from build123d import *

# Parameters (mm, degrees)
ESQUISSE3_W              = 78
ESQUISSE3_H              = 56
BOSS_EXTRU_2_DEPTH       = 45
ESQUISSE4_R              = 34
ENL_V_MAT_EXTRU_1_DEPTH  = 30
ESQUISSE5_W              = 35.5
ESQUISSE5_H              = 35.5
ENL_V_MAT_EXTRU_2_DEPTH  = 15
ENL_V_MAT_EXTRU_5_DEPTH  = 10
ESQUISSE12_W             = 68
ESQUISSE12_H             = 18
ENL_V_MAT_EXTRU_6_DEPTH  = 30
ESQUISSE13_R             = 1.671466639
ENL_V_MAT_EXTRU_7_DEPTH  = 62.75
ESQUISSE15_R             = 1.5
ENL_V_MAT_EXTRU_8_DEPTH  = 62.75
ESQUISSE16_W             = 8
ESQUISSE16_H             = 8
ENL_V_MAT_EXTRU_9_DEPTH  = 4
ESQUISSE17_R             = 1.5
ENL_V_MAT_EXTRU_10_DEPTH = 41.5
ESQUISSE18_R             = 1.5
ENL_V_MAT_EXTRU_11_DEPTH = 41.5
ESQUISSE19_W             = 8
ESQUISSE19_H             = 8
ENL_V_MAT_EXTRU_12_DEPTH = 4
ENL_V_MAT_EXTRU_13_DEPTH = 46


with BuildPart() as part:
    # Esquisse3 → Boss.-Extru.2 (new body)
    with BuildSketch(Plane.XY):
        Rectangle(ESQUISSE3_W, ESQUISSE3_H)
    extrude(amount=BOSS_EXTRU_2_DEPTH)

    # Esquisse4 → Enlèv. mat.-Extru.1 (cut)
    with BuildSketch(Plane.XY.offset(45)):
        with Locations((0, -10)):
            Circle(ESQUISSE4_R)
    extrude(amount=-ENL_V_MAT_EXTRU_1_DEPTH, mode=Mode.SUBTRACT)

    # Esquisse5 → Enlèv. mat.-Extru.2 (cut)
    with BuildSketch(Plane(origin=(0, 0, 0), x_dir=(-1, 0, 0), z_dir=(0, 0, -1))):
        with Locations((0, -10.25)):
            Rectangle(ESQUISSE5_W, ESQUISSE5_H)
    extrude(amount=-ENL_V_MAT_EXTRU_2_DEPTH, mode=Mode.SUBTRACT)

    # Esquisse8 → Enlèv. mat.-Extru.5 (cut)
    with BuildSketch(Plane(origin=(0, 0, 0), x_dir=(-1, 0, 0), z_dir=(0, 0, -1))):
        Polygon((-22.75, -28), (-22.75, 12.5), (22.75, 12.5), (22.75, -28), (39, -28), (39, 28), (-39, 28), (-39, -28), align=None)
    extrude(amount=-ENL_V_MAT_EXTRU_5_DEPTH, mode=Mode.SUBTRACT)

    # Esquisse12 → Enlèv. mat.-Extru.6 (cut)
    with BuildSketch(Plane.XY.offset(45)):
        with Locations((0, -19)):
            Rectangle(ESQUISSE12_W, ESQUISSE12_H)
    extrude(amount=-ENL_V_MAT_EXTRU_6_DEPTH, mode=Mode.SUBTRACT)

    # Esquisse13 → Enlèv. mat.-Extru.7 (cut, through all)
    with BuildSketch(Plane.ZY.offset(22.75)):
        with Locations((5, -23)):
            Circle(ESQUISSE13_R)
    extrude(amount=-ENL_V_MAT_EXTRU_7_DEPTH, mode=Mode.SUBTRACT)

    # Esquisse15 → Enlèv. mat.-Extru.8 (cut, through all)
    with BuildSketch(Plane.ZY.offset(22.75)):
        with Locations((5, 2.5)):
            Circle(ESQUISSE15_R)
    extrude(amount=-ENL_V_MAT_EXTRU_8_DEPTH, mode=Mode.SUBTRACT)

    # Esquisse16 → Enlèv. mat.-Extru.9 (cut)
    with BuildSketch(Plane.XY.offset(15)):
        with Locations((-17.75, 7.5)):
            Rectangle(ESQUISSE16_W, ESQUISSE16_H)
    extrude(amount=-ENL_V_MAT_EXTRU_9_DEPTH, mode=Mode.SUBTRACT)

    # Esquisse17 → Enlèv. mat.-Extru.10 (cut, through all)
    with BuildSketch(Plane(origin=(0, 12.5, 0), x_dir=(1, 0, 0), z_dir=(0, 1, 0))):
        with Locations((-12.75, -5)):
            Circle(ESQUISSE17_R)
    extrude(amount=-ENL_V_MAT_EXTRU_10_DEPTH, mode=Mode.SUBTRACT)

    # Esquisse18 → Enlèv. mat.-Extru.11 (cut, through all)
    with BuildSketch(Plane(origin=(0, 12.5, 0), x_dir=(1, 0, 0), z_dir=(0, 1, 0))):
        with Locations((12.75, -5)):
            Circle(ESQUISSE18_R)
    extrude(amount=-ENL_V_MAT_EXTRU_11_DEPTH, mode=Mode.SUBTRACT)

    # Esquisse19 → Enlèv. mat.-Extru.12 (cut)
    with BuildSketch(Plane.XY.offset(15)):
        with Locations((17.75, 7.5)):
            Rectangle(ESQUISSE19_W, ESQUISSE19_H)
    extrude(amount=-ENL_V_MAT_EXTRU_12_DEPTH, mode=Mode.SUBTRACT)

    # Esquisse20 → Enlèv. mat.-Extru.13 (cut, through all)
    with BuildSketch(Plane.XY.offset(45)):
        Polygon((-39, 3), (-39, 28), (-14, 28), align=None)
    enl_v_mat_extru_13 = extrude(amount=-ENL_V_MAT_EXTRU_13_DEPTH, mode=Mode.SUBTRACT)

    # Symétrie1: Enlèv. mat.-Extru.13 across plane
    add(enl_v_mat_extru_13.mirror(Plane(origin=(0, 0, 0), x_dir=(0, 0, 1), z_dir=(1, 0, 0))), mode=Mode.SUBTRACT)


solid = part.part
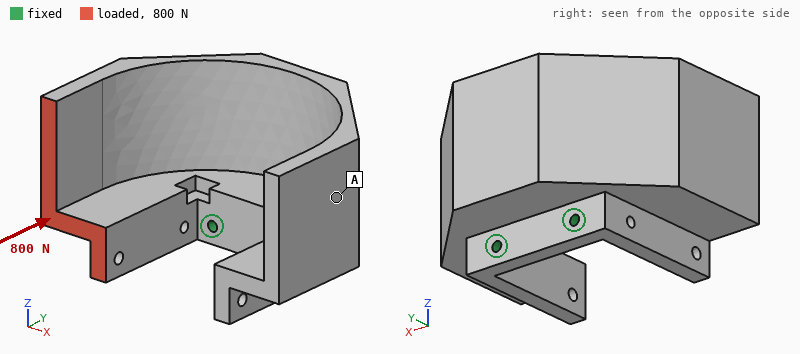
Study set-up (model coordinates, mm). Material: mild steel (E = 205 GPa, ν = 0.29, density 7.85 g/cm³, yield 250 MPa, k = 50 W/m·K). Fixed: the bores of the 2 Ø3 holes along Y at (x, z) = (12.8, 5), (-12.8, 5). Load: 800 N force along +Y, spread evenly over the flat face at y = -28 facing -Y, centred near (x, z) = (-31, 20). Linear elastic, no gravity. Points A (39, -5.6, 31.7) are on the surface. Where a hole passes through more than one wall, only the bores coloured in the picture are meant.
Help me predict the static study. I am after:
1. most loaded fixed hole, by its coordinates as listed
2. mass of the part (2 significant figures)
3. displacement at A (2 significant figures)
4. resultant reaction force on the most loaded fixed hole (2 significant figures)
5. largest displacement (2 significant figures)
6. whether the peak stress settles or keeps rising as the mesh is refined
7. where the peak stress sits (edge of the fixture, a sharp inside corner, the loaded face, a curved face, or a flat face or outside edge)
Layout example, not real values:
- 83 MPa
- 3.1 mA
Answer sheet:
- (-12.8, 5)
- 300 g
- 0.020 mm
- 1.3 kN
- 0.11 mm
- keeps rising
- edge of the fixture
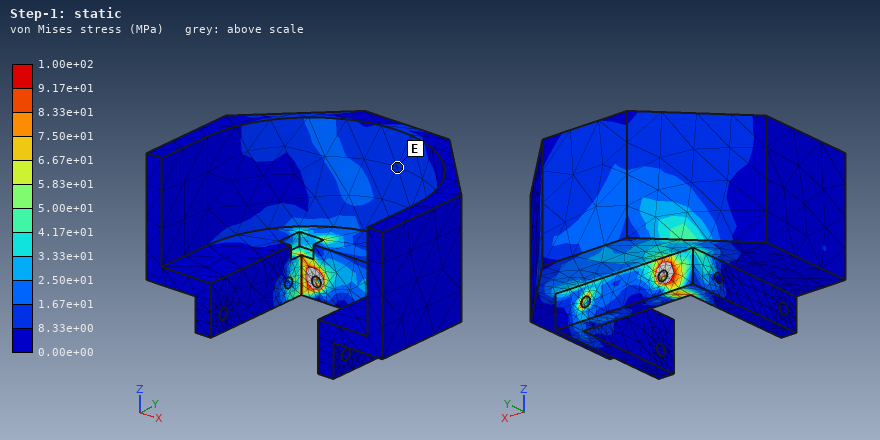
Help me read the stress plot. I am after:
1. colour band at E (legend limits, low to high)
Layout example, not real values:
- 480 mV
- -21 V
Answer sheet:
- 8.33e+00 to 1.67e+01 MPa
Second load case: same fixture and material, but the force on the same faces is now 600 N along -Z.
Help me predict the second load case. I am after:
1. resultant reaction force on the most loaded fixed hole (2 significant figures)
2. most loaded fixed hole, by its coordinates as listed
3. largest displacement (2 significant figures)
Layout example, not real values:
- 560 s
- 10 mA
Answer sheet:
- 1.0 kN
- (-12.8, 5)
- 0.16 mm
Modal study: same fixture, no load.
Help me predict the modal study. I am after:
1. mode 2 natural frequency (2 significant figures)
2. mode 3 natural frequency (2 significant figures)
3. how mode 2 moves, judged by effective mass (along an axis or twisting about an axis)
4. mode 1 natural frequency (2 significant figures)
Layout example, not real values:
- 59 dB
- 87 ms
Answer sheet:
- 1300 Hz
- 1600 Hz
- along X
- 1200 Hz
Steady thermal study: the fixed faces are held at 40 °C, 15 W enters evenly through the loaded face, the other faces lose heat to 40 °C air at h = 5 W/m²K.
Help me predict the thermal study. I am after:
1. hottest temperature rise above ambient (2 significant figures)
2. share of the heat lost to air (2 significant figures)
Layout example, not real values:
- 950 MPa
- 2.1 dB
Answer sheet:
- 71 K
- 14 %
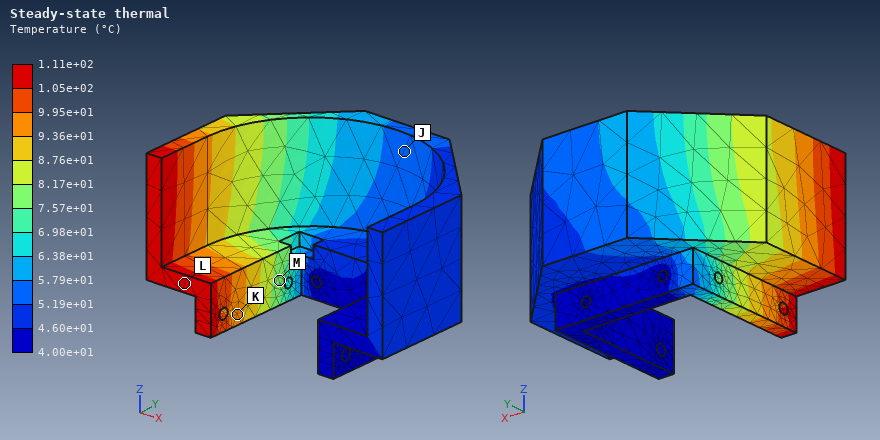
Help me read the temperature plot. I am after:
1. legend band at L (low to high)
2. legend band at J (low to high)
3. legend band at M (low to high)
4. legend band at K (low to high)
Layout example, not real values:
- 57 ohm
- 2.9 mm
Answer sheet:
- 1.05e+02 to 1.11e+02 °C
- 5.19e+01 to 5.79e+01 °C
- 7.57e+01 to 8.17e+01 °C
- 9.36e+01 to 9.95e+01 °C
